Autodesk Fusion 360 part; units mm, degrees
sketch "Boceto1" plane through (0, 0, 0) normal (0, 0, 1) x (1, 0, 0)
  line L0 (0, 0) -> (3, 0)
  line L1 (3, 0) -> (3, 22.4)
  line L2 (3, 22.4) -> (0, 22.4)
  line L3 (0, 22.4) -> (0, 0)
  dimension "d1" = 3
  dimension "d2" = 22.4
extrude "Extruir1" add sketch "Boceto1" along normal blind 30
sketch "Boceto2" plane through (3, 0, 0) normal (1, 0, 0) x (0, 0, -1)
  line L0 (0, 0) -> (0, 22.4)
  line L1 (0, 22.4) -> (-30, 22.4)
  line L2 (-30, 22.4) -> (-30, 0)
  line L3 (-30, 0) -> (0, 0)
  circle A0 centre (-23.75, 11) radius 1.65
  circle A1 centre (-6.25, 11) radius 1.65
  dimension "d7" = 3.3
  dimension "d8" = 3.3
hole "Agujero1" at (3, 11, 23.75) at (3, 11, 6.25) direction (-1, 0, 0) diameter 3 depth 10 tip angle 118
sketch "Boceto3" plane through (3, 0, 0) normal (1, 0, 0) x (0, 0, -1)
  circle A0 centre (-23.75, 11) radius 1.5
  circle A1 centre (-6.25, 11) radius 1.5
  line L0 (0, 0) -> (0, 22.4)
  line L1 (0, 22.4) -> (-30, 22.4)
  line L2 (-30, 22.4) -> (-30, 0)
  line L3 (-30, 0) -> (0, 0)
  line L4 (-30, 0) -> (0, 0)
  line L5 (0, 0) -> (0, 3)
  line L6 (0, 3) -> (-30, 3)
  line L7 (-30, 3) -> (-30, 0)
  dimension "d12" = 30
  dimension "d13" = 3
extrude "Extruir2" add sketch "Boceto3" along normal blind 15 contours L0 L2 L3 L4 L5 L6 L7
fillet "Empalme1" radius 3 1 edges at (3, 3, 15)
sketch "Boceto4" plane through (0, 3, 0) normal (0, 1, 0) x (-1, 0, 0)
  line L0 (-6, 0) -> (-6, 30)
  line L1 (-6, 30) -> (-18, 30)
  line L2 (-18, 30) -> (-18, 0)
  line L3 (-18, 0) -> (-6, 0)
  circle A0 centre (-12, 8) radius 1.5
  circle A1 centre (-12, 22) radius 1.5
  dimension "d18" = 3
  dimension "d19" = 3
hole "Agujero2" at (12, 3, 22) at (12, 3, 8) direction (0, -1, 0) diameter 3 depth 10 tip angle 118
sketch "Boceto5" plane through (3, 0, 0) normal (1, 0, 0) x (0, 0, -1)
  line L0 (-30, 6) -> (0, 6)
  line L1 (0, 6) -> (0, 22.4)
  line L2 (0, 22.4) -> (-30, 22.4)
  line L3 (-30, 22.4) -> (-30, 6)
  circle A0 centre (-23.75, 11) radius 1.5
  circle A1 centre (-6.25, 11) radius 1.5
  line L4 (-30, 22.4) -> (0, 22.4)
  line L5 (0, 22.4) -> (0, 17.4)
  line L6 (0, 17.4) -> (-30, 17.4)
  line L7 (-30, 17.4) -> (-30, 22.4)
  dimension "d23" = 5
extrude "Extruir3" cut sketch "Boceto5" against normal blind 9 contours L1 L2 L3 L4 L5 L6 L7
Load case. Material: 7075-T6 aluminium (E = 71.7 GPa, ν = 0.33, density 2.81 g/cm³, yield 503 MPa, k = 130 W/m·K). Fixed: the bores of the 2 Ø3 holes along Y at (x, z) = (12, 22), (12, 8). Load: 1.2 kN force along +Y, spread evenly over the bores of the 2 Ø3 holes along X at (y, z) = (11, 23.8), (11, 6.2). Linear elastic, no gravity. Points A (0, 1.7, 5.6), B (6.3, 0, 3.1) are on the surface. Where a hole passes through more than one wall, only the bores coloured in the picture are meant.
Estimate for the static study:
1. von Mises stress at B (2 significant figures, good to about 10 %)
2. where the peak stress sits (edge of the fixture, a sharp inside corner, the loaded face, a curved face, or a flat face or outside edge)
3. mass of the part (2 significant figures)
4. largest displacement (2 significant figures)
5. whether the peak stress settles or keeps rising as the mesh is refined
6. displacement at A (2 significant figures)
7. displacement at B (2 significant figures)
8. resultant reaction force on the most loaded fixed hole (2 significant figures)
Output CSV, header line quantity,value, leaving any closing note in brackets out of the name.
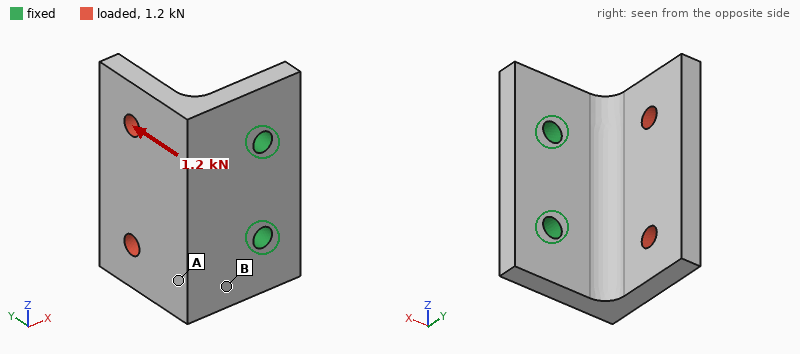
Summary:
quantity,value
von Mises stress at B,110 MPa
where the peak stress sits,edge of the fixture
mass of the part,8.1 g
largest displacement,0.24 mm
whether the peak stress settles or keeps rising as the mesh is refined,keeps rising
displacement at A,0.12 mm
displacement at B,0.044 mm
resultant reaction force on the most loaded fixed hole,600 N
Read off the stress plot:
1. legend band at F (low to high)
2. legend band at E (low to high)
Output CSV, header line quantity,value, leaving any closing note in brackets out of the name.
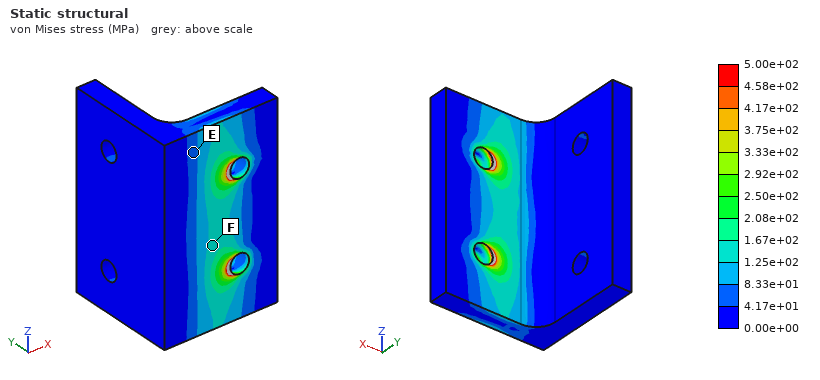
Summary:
quantity,value
legend band at F,1.25e+02 to 1.67e+02 MPa
legend band at E,4.17e+01 to 8.33e+01 MPa
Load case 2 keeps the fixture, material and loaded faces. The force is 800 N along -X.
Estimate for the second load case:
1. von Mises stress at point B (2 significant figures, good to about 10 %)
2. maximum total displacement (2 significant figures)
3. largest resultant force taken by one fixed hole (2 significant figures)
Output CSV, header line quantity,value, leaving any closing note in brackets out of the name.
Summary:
quantity,value
von Mises stress at point B,140 MPa
maximum total displacement,0.28 mm
largest resultant force taken by one fixed hole,400 N
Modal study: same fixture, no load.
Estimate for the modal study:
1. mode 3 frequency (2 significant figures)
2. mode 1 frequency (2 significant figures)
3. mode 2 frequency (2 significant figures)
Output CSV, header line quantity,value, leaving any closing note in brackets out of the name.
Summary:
quantity,value
mode 3 frequency,15 kHz
mode 1 frequency,5000 Hz
mode 2 frequency,8300 Hz
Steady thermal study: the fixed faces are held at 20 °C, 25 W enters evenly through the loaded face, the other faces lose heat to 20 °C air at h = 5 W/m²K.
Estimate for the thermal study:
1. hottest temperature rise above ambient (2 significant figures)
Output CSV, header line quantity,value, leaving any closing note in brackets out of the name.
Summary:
quantity,value
hottest temperature rise above ambient,45 K
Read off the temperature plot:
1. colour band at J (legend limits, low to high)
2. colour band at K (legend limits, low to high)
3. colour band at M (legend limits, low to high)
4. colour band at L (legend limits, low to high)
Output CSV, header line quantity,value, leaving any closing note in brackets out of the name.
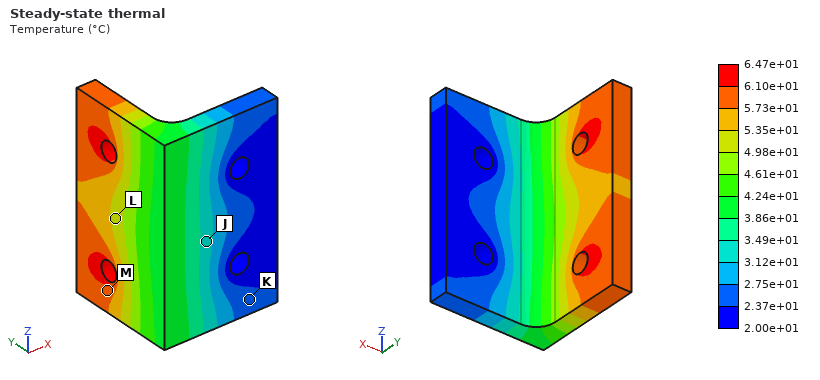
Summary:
quantity,value
colour band at J,3.12e+01 to 3.49e+01 °C
colour band at K,2.37e+01 to 2.75e+01 °C
colour band at M,5.73e+01 to 6.10e+01 °C
colour band at L,4.98e+01 to 5.35e+01 °C
